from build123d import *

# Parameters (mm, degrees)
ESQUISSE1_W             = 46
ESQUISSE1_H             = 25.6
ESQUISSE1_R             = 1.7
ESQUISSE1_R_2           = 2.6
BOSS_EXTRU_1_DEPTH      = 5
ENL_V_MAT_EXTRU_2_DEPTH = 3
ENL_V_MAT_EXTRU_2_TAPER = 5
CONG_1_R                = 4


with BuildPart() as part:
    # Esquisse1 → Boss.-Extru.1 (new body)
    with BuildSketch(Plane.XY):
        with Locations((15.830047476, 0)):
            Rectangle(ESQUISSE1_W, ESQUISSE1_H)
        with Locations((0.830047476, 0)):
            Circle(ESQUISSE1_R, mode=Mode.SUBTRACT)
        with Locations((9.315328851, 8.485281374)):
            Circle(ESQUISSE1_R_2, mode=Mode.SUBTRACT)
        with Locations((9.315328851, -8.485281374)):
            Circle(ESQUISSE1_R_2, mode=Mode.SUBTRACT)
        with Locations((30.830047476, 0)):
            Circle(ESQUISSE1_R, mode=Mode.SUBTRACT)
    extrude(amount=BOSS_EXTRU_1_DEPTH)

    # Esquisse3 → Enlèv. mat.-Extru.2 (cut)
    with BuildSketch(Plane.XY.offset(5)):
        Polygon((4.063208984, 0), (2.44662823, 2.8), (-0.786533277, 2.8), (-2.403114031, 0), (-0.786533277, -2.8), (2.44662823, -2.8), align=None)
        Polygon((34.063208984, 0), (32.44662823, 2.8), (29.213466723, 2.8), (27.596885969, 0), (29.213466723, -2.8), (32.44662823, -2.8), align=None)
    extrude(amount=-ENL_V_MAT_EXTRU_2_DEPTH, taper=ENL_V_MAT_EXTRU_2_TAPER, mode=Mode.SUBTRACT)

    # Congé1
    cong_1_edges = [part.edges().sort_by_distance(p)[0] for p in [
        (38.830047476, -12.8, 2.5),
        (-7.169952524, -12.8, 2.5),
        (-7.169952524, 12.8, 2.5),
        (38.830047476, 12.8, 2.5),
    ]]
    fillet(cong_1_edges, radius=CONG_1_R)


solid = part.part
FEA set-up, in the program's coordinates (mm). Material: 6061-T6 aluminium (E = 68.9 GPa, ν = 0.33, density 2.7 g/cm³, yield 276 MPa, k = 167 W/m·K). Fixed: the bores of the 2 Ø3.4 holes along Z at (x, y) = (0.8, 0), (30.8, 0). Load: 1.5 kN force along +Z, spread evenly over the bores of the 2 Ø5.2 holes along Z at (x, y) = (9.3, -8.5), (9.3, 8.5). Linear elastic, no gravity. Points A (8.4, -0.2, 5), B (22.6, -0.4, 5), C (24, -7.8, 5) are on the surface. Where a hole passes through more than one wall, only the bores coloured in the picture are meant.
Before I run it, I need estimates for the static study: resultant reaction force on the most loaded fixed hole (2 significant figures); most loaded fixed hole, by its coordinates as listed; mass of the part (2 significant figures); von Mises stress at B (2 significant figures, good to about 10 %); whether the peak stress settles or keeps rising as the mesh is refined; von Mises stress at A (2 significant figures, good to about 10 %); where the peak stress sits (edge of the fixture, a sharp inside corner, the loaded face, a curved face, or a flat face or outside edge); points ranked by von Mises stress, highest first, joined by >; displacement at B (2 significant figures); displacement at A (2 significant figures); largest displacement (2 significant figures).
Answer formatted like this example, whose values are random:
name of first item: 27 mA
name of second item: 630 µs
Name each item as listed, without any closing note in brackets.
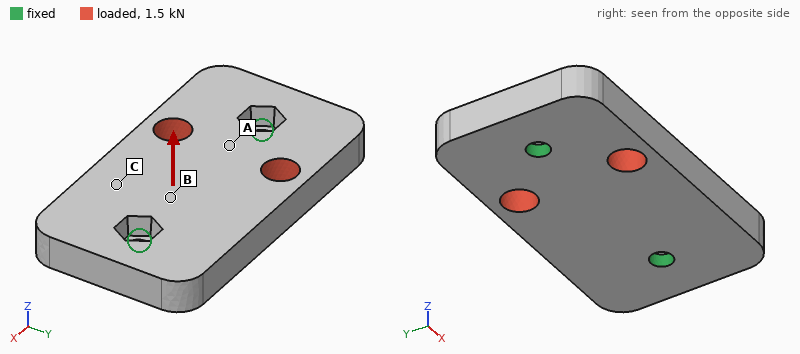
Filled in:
resultant reaction force on the most loaded fixed hole: 1.4 kN
most loaded fixed hole, by its coordinates as listed: (0.8, 0)
mass of the part: 15 g
von Mises stress at B: 34 MPa
whether the peak stress settles or keeps rising as the mesh is refined: keeps rising
von Mises stress at A: 81 MPa
where the peak stress sits: edge of the fixture
points ranked by von Mises stress, highest first, joined by >: A > B > C
displacement at B: 16 µm
displacement at A: 22 µm
largest displacement: 44 µm
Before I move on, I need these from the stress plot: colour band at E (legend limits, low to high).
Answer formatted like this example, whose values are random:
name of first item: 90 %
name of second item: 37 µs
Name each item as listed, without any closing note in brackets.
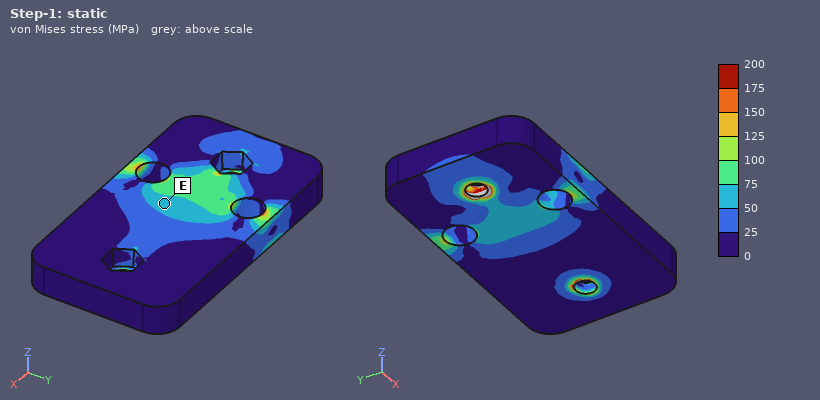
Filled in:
colour band at E: 50 to 75 MPa
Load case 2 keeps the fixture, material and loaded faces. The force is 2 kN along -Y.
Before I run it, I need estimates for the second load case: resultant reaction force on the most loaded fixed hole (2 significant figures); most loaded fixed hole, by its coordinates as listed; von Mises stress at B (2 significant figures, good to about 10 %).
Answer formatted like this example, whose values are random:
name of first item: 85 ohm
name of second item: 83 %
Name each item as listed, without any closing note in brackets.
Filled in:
resultant reaction force on the most loaded fixed hole: 1.4 kN
most loaded fixed hole, by its coordinates as listed: (0.8, 0)
von Mises stress at B: 20 MPa
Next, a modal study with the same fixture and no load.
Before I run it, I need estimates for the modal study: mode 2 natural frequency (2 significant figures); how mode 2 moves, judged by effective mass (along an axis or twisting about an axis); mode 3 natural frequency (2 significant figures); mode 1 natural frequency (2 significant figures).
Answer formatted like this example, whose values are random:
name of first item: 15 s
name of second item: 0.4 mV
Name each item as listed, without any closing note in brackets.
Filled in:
mode 2 natural frequency: 14 kHz
how mode 2 moves, judged by effective mass: along Z
mode 3 natural frequency: 15 kHz
mode 1 natural frequency: 7400 Hz
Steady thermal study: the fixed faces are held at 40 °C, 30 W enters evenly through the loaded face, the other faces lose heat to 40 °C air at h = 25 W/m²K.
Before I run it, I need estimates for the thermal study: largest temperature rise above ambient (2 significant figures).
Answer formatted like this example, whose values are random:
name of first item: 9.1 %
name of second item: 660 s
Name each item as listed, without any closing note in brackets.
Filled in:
largest temperature rise above ambient: 18 K
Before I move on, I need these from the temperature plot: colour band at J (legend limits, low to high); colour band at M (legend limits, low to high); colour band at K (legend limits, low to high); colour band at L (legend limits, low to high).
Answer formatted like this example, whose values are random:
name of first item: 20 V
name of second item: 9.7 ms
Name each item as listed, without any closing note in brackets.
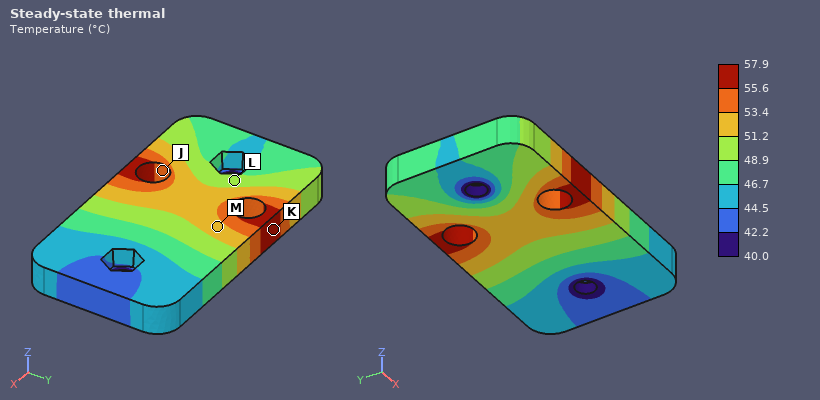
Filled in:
colour band at J: 53.4 to 55.6 °C
colour band at M: 51.2 to 53.4 °C
colour band at K: 55.6 to 57.9 °C
colour band at L: 48.9 to 51.2 °C
